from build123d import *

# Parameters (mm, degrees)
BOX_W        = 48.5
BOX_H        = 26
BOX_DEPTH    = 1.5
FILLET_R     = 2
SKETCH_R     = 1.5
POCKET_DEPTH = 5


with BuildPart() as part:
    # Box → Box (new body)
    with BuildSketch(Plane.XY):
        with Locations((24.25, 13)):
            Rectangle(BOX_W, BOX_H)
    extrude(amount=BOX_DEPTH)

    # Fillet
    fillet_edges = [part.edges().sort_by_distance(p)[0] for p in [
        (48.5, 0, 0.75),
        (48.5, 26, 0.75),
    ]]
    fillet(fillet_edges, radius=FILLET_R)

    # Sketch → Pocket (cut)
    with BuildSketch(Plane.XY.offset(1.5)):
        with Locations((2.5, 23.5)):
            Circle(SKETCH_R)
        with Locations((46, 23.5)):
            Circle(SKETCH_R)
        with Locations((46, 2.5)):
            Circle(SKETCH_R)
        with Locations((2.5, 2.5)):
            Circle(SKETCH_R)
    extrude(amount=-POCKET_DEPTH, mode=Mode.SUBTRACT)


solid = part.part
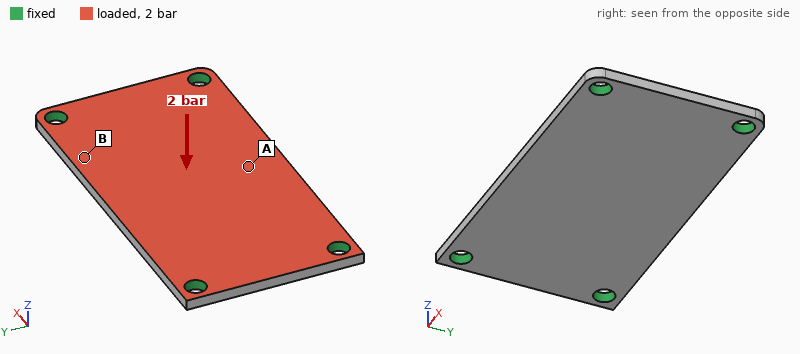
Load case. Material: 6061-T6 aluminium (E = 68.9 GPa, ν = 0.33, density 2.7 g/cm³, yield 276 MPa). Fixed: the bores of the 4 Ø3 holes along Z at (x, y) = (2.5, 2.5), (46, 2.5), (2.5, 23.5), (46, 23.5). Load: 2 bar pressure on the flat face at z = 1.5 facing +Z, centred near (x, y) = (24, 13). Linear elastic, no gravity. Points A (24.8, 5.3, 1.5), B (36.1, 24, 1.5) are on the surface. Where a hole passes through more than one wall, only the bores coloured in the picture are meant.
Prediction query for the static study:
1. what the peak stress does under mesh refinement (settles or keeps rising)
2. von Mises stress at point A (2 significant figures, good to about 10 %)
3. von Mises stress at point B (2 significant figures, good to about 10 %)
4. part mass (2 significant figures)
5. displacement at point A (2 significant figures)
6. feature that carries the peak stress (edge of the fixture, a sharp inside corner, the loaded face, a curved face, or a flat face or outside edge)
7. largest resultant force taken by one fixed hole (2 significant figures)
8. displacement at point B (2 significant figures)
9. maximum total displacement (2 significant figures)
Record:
keeps rising
40 MPa
14 MPa
5.0 g
0.099 mm
edge of the fixture
62 N
0.048 mm
0.10 mm
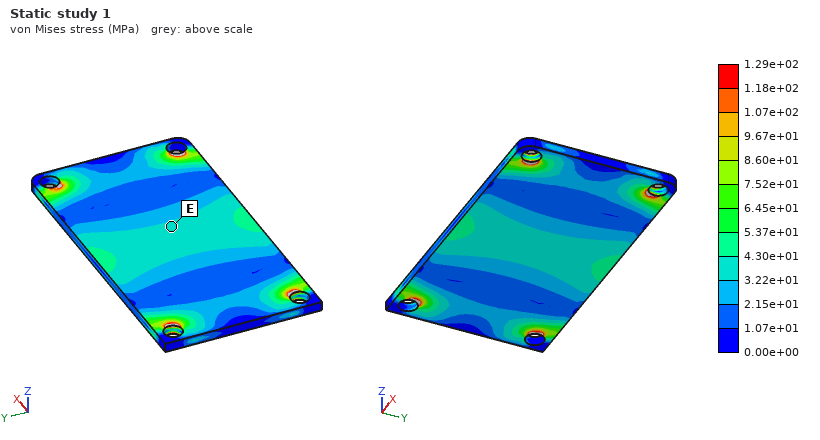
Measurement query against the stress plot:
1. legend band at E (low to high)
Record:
3.22e+01 to 4.30e+01 MPa
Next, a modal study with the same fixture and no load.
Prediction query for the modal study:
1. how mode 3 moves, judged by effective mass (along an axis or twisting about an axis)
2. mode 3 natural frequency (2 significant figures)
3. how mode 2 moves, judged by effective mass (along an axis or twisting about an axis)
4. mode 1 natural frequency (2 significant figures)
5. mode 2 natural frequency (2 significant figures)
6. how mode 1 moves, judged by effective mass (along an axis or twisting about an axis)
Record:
twisting about Y
11 kHz
twisting about X
4000 Hz
6500 Hz
along Z
